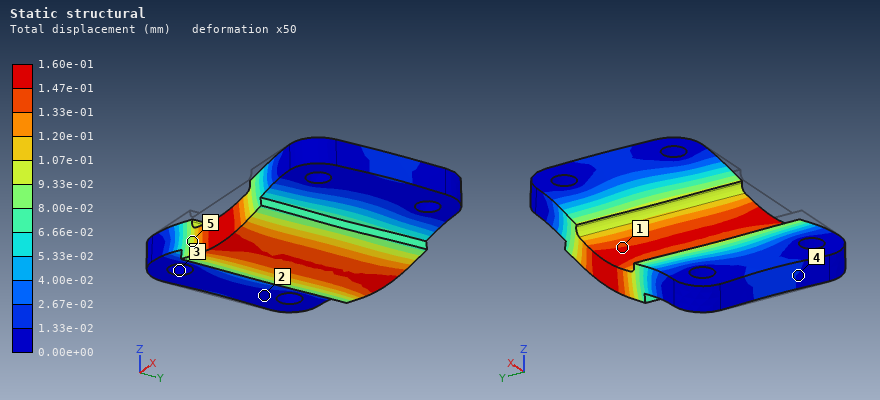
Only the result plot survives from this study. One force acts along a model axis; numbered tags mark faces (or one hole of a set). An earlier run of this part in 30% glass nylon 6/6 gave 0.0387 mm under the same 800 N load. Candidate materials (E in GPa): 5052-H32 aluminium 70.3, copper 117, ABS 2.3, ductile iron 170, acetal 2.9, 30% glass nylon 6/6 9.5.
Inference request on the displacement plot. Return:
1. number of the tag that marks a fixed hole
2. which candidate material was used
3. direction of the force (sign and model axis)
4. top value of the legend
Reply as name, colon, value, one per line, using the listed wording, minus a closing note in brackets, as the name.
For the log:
number of the tag that marks a fixed hole: 3
which candidate material was used: ABS
direction of the force: -Z
top value of the legend: 1.60e-01 mm
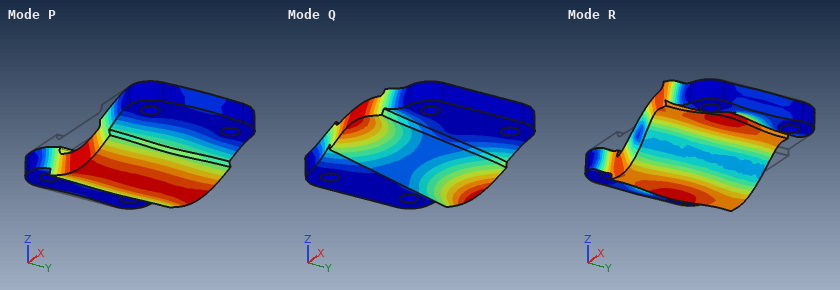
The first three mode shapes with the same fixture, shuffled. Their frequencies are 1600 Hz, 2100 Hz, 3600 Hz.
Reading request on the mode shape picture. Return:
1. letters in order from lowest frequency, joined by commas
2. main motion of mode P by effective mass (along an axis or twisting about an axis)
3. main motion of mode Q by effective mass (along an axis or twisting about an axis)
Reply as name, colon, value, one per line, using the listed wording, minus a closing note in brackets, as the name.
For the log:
letters in order from lowest frequency, joined by commas: P, Q, R
main motion of mode P by effective mass: along Z
main motion of mode Q by effective mass: twisting about X
